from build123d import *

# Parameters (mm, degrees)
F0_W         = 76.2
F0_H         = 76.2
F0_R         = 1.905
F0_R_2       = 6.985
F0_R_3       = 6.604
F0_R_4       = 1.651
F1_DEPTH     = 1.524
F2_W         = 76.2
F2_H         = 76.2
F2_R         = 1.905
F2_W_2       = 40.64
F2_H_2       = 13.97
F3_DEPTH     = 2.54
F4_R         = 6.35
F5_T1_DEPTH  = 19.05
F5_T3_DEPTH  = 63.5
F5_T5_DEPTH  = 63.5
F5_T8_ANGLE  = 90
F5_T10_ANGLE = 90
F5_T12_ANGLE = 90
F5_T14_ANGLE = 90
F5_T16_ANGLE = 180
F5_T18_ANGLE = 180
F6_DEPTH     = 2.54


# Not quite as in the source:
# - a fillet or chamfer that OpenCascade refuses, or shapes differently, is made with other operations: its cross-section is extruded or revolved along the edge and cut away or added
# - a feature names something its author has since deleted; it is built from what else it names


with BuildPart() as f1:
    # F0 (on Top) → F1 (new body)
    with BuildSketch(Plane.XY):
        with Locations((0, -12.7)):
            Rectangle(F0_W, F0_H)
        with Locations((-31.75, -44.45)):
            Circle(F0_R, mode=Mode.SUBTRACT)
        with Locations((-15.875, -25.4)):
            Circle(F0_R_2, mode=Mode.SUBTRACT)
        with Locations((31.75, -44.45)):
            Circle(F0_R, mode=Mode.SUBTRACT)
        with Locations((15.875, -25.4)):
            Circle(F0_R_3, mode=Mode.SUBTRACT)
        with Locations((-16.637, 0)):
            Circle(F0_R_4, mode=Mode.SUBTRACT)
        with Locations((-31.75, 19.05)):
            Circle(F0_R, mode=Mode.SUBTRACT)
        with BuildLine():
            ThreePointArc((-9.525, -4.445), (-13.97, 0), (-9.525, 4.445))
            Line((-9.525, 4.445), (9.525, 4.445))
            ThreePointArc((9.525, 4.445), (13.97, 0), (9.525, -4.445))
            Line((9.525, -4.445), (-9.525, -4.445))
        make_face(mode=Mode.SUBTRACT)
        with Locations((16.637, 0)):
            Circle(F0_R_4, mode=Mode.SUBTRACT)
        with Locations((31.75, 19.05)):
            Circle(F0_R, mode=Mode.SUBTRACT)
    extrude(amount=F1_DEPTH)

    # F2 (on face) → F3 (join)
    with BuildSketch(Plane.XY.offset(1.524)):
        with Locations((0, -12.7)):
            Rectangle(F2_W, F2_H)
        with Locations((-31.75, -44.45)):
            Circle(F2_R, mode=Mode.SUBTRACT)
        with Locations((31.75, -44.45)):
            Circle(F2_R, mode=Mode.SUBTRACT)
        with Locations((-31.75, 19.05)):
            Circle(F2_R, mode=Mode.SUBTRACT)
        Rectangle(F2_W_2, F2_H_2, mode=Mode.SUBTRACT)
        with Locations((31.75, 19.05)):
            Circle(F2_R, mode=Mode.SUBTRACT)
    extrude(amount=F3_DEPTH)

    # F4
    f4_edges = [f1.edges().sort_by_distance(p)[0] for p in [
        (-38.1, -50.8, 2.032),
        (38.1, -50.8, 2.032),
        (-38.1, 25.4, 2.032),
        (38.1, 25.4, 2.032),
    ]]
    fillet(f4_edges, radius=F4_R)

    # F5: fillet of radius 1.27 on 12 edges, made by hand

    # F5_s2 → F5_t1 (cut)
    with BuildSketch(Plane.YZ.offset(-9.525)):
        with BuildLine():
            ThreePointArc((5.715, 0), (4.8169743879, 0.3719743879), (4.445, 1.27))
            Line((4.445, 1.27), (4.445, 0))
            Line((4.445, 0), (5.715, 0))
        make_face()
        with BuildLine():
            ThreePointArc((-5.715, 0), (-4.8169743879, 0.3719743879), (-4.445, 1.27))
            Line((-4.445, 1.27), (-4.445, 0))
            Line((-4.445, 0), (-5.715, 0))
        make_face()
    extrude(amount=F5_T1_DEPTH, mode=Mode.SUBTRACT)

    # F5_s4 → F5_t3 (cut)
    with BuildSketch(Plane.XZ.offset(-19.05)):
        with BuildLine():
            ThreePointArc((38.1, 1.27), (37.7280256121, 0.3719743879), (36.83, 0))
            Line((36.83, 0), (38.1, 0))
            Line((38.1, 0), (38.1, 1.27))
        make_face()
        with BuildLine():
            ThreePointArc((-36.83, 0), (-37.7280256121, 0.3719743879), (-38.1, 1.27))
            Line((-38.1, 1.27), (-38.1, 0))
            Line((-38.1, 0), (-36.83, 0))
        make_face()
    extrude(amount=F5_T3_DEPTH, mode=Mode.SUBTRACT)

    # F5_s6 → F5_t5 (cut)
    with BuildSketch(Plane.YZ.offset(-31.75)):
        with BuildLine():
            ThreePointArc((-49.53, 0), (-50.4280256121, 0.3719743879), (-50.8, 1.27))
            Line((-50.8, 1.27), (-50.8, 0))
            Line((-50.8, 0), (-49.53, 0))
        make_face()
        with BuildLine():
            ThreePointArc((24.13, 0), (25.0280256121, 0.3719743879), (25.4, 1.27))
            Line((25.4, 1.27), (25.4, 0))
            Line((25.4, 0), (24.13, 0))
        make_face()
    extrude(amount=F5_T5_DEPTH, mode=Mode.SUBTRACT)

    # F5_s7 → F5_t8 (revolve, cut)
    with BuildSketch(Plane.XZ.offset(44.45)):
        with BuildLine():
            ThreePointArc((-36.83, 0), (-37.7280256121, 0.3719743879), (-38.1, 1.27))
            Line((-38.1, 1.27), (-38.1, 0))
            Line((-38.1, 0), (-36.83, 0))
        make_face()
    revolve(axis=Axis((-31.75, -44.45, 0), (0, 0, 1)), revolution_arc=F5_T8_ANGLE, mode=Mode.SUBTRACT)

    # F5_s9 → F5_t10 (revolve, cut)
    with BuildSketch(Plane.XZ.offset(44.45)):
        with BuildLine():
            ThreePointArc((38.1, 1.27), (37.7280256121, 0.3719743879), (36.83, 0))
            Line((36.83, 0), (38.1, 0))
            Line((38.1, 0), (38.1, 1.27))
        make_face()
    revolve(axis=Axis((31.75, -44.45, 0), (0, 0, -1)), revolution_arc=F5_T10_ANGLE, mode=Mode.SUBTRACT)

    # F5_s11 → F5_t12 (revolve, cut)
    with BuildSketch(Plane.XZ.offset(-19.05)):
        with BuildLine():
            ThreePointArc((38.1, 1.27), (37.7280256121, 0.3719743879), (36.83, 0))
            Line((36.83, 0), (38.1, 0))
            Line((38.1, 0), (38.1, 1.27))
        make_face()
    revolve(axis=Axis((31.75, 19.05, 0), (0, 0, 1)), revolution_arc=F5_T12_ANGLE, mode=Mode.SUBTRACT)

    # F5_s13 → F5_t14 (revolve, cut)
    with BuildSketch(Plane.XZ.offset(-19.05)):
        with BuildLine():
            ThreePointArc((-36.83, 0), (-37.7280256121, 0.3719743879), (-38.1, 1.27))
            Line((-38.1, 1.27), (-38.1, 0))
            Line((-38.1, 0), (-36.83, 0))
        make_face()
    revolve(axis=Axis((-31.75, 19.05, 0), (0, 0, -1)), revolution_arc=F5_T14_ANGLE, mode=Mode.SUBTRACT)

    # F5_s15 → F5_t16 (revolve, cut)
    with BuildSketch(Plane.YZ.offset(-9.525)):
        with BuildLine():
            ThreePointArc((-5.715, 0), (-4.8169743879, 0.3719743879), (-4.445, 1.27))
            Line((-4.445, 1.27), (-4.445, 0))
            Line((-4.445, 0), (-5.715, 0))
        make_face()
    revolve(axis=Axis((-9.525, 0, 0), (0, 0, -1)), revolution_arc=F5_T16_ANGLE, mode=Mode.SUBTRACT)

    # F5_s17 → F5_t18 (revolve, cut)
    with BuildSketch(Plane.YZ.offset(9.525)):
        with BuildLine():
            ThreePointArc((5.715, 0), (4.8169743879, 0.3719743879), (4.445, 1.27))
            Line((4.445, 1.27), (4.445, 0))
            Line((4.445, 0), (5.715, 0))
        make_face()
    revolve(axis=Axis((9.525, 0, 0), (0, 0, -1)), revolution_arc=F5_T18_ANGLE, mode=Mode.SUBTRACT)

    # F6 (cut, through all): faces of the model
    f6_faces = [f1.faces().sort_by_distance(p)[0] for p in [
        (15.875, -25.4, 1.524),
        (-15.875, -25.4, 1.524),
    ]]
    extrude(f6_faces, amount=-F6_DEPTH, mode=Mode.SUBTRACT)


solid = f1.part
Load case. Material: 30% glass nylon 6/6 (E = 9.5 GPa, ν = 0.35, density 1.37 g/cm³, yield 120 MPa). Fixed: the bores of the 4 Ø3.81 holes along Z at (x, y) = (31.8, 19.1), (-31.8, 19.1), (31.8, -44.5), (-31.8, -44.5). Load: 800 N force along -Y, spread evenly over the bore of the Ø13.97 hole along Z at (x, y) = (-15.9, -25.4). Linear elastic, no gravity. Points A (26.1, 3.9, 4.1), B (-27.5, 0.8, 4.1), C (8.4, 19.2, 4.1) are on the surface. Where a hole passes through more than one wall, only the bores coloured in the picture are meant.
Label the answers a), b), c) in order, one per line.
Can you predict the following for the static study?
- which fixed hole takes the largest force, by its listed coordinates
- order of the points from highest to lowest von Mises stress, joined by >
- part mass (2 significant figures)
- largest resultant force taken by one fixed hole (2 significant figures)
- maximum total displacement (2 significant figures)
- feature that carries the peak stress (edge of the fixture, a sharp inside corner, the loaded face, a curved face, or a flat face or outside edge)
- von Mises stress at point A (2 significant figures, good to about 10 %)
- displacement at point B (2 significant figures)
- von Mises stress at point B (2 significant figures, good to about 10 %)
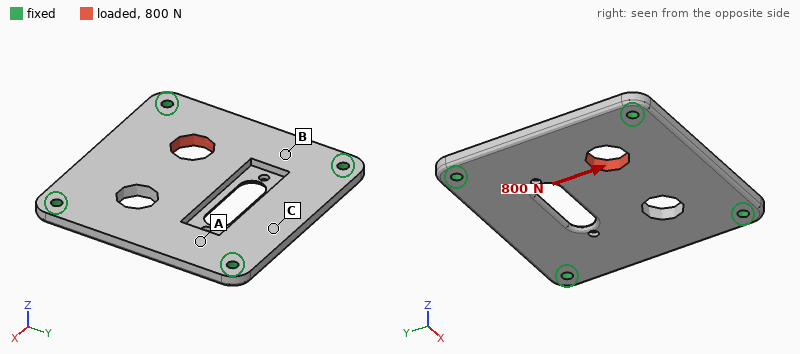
a) (-31.8, -44.5)
b) B > A > C
c) 28 g
d) 390 N
e) 27 µm
f) a curved face
g) 1.9 MPa
h) 8.3 µm
i) 3.7 MPa
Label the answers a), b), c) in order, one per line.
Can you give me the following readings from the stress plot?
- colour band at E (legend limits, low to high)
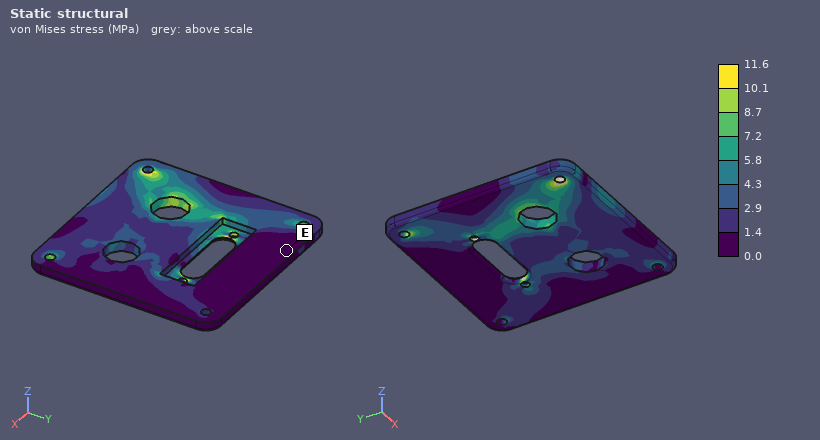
a) 0.0 to 1.4 MPa
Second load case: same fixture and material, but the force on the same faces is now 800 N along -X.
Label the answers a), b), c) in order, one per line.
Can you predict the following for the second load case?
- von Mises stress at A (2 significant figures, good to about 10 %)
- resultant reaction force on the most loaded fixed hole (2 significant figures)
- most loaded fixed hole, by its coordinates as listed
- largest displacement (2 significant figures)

a) 2.0 MPa
b) 380 N
c) (-31.8, -44.5)
d) 30 µm
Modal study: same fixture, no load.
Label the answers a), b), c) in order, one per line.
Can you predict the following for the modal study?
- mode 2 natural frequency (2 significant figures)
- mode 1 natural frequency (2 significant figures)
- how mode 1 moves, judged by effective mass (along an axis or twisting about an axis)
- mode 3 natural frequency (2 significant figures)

a) 2800 Hz
b) 1700 Hz
c) along Z
d) 2900 Hz
